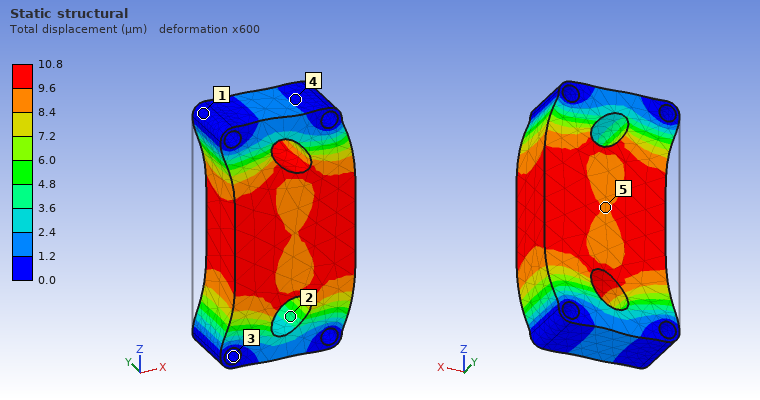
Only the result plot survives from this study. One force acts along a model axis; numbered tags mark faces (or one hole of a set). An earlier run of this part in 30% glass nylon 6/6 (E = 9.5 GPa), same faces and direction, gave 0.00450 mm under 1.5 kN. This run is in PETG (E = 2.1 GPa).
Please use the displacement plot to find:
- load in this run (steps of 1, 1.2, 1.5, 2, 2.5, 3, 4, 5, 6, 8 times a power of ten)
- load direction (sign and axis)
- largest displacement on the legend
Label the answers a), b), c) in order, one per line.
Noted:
a) 800 N
b) +X
c) 10.8 µm
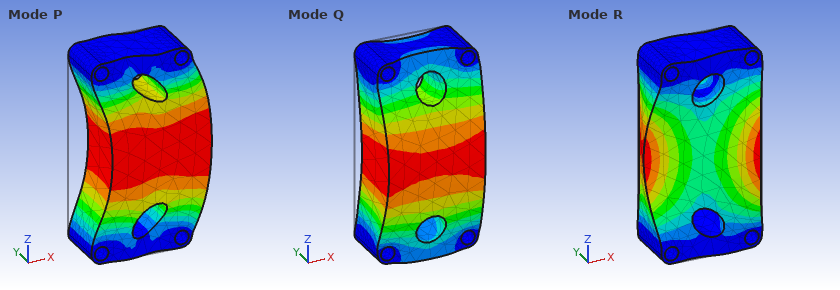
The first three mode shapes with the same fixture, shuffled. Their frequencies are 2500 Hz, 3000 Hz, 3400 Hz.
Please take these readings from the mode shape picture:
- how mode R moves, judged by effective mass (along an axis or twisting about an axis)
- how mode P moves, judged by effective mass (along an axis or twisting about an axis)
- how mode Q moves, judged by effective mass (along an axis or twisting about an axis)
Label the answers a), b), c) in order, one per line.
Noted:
a) twisting about Z
b) along X
c) along Y
